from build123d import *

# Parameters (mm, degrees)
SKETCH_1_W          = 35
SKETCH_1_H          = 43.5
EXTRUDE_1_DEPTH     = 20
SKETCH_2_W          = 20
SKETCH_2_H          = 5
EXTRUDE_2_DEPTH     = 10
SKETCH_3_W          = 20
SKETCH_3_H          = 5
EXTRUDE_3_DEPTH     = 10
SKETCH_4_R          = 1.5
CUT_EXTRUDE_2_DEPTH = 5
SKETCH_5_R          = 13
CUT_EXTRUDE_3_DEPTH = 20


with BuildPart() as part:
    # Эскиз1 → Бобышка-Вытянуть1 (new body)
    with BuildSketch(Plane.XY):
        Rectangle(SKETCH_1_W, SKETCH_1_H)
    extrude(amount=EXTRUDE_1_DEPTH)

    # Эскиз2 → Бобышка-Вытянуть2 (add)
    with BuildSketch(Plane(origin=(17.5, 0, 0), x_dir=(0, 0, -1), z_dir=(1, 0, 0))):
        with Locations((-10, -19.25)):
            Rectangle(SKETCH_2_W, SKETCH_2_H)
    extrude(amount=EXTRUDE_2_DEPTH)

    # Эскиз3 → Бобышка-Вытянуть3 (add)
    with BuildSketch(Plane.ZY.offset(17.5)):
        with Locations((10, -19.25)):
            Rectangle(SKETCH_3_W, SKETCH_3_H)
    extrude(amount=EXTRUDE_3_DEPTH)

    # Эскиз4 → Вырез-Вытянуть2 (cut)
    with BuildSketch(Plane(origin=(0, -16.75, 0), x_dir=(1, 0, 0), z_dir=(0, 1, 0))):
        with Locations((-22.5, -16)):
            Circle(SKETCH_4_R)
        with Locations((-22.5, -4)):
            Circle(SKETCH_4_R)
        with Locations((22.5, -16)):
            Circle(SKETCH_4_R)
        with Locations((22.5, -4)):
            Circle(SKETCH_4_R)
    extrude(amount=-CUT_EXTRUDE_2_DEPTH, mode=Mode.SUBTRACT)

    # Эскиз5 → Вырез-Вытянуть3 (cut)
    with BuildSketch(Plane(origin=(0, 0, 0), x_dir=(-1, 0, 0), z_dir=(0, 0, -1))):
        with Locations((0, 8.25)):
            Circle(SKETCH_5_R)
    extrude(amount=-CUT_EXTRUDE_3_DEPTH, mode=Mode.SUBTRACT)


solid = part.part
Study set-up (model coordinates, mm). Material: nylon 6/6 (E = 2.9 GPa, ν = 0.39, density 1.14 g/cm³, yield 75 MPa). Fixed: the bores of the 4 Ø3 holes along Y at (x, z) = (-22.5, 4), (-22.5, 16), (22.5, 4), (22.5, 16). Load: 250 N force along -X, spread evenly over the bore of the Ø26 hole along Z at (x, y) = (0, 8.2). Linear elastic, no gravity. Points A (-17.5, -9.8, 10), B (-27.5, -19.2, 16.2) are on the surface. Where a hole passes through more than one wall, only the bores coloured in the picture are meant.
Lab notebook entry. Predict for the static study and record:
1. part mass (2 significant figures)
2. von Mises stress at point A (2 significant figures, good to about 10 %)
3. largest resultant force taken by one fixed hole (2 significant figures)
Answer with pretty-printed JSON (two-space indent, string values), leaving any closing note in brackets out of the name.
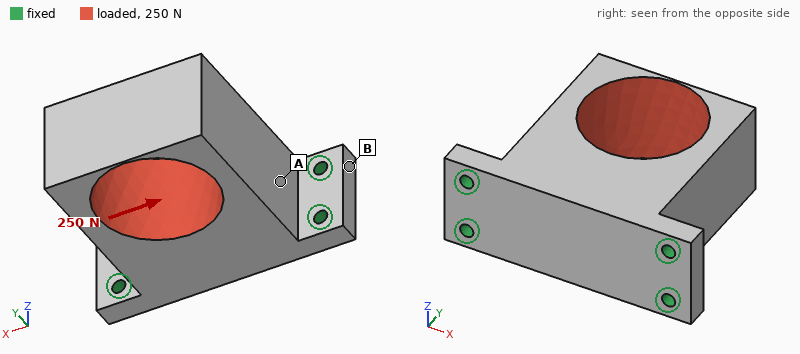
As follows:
{
  "part mass": "25 g",
  "von Mises stress at point A": "2.9 MPa",
  "largest resultant force taken by one fixed hole": "110 N"
}
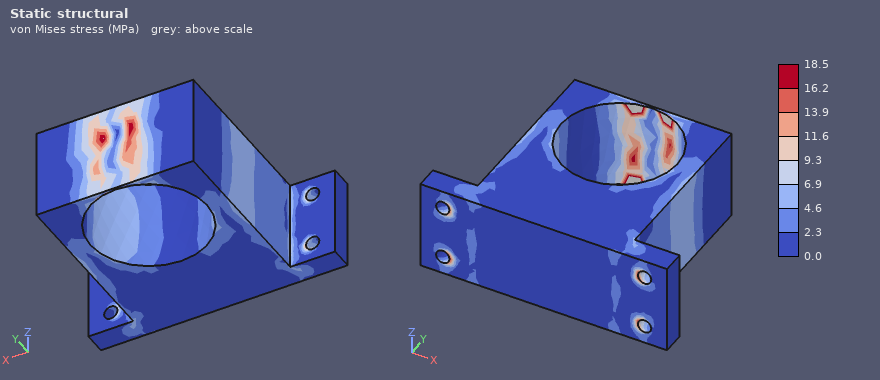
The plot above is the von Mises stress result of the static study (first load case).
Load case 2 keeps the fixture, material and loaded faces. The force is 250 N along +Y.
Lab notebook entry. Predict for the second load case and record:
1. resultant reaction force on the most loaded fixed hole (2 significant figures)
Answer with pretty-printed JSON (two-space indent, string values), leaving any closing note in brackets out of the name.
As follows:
{
  "resultant reaction force on the most loaded fixed hole": "68 N"
}
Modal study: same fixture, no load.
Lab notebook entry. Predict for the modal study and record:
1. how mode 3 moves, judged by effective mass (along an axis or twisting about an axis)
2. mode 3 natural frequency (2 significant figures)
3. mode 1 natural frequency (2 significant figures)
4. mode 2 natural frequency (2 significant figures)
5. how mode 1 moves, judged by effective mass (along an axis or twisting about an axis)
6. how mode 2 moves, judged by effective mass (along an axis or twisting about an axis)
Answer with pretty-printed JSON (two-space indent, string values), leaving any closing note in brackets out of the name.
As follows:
{
  "how mode 3 moves, judged by effective mass": "twisting about Y",
  "mode 3 natural frequency": "3200 Hz",
  "mode 1 natural frequency": "1200 Hz",
  "mode 2 natural frequency": "1800 Hz",
  "how mode 1 moves, judged by effective mass": "along Z",
  "how mode 2 moves, judged by effective mass": "along X"
}
